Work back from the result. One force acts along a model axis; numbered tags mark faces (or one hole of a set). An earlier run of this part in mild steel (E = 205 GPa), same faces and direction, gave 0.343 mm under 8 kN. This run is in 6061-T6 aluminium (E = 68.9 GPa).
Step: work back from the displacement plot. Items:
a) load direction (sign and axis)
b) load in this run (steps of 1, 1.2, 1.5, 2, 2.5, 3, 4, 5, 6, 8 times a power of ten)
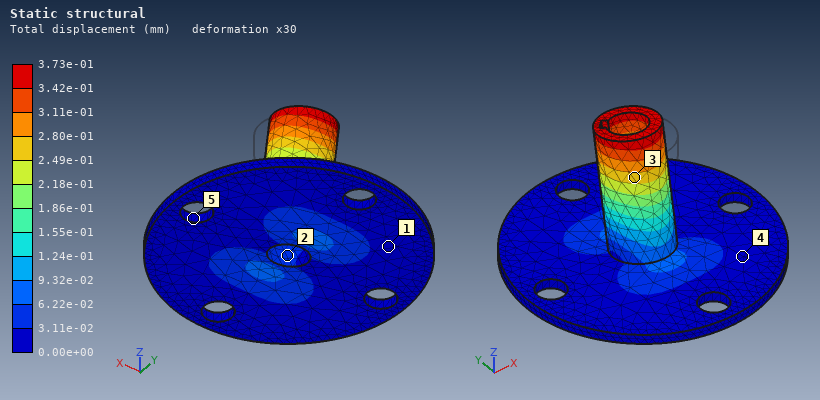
+Y
3 kN
